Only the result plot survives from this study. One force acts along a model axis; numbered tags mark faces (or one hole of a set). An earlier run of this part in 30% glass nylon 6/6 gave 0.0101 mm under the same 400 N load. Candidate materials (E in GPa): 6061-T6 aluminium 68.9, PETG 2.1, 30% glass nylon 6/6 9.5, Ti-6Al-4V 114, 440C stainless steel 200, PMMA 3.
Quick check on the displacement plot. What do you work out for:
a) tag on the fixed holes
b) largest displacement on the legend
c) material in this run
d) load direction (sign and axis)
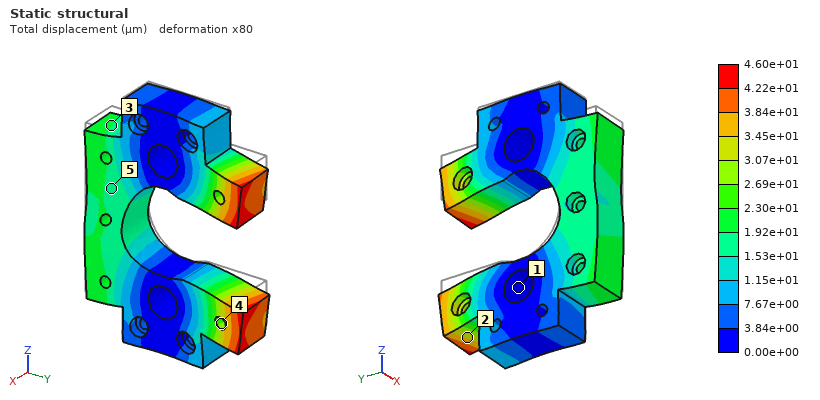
1
4.60e+01 µm
PETG
-Z
